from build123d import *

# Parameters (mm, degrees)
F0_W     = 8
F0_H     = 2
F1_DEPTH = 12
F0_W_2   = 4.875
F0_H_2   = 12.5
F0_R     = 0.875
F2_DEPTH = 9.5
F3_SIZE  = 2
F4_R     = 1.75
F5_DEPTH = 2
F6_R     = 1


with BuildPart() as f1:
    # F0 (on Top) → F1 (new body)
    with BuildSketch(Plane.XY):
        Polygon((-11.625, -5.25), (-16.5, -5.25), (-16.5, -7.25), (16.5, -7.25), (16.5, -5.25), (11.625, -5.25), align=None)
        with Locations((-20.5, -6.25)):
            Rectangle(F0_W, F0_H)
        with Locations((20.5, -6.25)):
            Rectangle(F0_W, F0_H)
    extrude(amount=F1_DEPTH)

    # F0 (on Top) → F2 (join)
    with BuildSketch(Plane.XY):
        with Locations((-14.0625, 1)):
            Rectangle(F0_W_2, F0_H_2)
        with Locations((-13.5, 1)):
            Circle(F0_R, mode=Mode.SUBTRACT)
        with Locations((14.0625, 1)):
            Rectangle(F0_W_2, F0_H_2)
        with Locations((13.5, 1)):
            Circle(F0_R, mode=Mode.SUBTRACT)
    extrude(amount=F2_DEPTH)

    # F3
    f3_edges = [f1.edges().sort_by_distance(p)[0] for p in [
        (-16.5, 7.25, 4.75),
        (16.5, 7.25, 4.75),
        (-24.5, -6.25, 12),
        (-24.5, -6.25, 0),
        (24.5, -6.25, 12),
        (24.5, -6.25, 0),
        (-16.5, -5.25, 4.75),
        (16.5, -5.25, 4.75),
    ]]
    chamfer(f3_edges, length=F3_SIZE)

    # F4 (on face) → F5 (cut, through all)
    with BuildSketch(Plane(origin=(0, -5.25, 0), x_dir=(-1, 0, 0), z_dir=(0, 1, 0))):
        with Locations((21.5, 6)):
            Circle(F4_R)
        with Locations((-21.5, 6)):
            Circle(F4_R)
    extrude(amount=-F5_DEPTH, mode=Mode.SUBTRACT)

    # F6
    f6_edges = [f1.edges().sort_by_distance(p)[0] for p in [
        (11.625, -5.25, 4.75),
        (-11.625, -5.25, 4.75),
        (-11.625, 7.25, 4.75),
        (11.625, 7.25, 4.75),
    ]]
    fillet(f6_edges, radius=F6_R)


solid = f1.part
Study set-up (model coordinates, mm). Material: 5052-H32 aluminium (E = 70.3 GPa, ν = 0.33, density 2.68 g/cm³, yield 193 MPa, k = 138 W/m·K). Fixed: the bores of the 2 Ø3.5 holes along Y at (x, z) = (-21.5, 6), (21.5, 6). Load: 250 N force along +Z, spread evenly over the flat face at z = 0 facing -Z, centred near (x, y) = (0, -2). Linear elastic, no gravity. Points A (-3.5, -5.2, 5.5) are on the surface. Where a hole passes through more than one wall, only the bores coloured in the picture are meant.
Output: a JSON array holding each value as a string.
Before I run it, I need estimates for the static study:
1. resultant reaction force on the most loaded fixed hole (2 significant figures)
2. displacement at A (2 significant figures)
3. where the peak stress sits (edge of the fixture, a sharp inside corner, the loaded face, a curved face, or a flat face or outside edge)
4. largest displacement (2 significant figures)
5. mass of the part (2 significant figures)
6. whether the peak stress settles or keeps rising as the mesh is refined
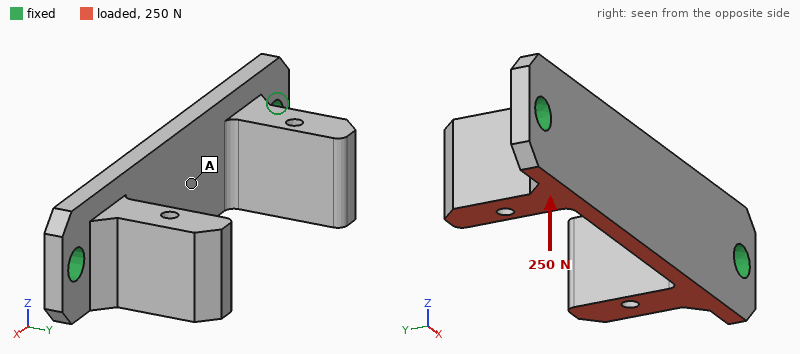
["130 N", "6.3 µm", "edge of the fixture", "24 µm", "6.0 g", "keeps rising"]
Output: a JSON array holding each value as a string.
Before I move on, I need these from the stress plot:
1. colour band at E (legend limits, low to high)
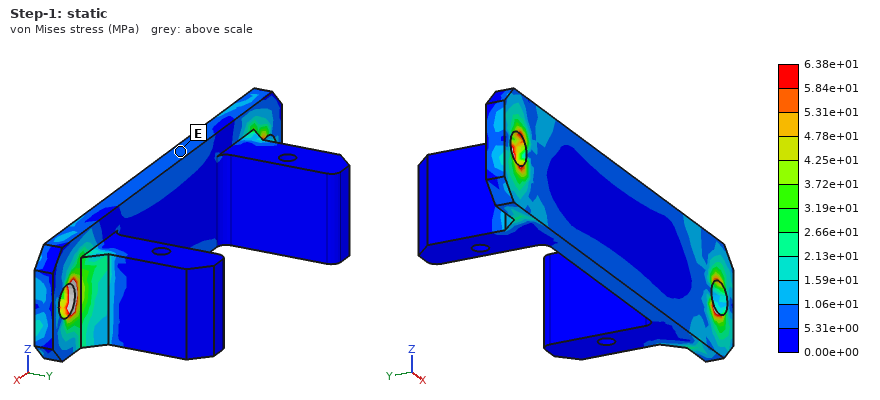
["5.31e+00 to 1.06e+01 MPa"]
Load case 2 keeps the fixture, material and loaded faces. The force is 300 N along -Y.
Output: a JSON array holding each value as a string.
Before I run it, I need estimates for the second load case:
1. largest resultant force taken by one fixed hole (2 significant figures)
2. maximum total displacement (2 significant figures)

["150 N", "88 µm"]
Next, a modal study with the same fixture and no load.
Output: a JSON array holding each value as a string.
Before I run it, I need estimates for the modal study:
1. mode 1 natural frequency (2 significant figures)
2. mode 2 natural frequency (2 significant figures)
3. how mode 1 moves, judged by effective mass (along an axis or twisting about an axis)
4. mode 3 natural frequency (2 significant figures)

["4700 Hz", "8100 Hz", "along Y", "8400 Hz"]
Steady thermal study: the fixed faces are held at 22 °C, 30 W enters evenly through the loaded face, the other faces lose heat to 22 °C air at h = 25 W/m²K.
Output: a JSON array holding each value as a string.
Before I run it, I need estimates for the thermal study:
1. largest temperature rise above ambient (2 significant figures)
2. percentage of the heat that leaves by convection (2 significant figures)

["34 K", "3.7 %"]
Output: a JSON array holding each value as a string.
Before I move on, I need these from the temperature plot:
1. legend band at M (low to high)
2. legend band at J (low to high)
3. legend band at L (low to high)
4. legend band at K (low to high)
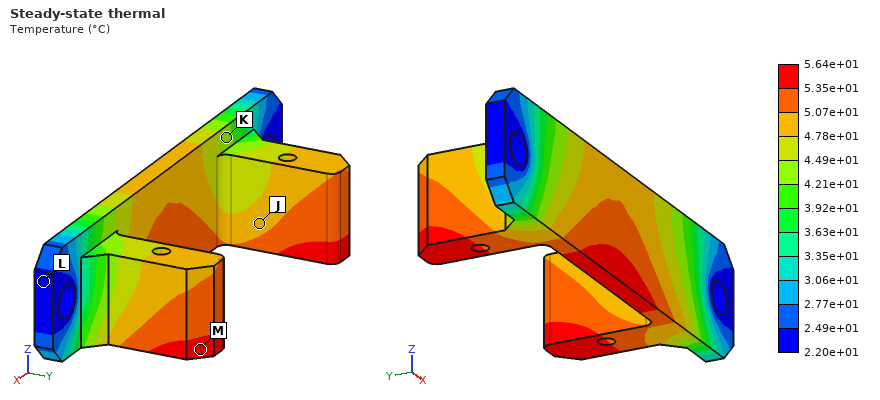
["5.35e+01 to 5.64e+01 °C", "4.78e+01 to 5.07e+01 °C", "2.20e+01 to 2.49e+01 °C", "4.21e+01 to 4.49e+01 °C"]
